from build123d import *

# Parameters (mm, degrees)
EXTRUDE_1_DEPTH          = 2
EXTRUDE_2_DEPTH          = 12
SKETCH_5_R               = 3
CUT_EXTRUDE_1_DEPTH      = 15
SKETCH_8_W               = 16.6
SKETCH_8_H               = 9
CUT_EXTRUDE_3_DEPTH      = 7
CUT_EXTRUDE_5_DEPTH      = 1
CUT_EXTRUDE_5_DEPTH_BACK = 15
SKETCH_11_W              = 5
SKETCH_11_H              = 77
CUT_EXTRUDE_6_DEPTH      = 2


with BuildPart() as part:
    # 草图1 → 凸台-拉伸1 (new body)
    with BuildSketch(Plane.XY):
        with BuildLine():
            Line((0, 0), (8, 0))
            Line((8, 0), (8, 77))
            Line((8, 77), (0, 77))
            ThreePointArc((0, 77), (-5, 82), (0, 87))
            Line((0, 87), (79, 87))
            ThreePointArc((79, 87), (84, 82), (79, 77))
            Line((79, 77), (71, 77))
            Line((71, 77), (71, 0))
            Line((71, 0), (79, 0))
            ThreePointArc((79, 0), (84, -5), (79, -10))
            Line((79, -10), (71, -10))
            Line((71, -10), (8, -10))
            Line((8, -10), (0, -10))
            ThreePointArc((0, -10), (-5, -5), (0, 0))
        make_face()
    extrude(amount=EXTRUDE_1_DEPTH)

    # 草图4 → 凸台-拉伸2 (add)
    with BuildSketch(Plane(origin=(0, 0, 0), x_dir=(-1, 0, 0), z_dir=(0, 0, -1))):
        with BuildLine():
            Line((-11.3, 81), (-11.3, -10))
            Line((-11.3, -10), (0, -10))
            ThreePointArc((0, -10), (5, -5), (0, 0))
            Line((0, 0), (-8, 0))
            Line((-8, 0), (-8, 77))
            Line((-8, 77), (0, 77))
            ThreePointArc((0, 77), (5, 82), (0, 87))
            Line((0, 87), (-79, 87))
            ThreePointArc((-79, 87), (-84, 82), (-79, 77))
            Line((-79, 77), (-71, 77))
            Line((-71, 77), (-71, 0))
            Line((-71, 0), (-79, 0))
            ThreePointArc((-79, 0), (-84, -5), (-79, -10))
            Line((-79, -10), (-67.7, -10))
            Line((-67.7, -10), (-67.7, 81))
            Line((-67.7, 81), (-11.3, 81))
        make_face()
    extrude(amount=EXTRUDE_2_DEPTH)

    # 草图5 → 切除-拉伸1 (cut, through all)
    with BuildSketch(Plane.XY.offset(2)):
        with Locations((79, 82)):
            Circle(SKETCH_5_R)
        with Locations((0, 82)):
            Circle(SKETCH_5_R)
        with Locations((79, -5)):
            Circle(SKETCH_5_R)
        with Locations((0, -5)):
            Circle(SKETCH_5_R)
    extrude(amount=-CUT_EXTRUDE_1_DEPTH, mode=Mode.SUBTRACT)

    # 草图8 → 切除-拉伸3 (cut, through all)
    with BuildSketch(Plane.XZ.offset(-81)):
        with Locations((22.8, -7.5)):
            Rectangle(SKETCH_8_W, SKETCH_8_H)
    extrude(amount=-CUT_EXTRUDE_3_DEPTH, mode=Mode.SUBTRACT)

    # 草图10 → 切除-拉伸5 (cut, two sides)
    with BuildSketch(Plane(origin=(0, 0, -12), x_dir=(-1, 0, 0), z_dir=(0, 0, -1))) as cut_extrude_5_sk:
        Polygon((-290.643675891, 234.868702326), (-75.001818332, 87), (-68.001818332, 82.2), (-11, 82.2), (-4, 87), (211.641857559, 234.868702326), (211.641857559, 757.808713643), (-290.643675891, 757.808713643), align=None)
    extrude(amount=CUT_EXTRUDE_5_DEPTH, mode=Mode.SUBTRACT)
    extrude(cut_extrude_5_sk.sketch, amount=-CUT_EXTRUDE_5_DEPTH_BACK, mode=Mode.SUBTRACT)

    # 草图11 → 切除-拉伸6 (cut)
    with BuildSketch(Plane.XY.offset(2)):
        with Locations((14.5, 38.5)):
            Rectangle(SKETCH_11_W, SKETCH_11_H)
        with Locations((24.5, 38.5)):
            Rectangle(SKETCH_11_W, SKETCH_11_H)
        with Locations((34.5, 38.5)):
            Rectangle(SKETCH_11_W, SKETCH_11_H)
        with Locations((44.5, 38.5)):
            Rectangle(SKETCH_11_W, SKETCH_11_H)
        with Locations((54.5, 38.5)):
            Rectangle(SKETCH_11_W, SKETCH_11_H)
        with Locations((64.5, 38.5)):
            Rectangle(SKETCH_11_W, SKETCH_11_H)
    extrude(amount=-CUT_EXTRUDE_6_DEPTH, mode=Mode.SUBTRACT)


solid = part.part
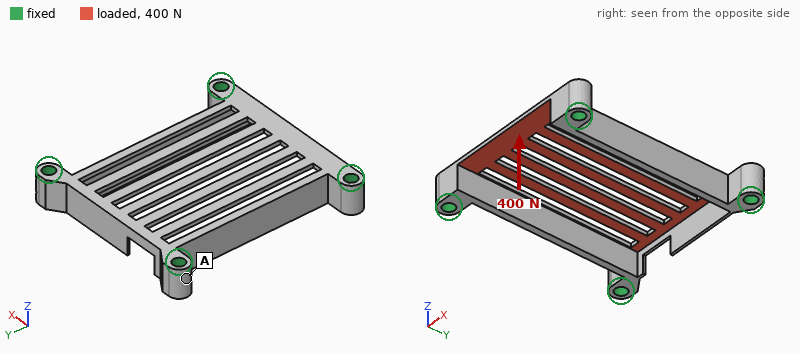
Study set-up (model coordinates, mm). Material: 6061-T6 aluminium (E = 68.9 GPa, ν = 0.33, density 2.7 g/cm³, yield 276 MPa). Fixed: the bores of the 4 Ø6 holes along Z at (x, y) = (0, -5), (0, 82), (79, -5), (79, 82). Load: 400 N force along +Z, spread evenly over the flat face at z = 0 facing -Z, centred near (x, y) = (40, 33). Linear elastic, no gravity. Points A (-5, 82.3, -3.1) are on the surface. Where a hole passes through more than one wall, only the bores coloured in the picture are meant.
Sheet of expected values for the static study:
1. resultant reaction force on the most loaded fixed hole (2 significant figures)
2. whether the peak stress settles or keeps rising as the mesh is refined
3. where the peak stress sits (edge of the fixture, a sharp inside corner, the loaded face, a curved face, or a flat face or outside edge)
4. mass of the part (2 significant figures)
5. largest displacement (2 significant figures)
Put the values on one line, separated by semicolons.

130 N; keeps rising; a sharp inside corner; 54 g; 1.0 mm
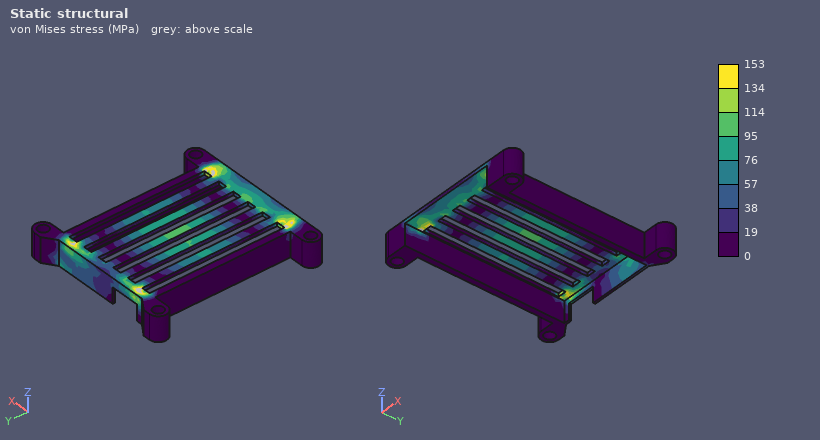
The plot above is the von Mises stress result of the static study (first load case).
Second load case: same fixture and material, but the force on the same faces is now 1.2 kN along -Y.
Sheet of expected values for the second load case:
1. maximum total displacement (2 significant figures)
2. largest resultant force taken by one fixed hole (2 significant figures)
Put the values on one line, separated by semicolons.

80 µm; 350 N
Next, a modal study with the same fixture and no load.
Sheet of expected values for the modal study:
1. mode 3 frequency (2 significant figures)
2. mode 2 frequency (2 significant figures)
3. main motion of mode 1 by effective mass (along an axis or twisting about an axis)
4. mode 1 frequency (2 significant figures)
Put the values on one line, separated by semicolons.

1400 Hz; 1300 Hz; along Z; 990 Hz
